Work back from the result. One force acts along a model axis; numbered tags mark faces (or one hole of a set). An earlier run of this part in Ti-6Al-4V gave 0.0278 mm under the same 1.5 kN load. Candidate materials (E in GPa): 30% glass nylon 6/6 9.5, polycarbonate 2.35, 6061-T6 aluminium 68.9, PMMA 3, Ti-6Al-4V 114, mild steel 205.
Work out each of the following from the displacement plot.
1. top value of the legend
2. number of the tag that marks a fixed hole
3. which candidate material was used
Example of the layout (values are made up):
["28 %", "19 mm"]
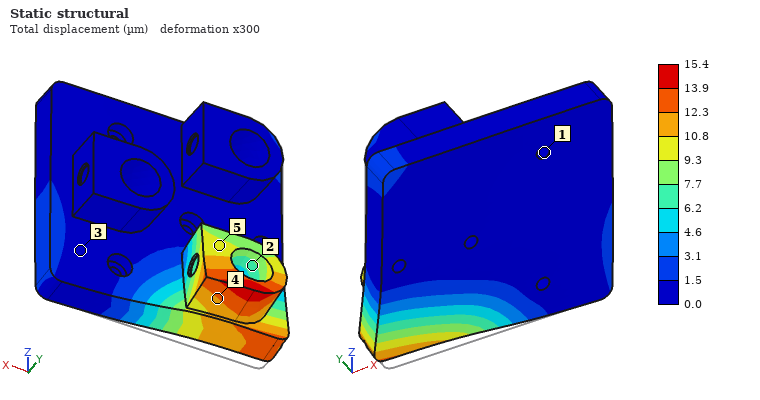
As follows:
["15.4 µm", "1", "mild steel"]
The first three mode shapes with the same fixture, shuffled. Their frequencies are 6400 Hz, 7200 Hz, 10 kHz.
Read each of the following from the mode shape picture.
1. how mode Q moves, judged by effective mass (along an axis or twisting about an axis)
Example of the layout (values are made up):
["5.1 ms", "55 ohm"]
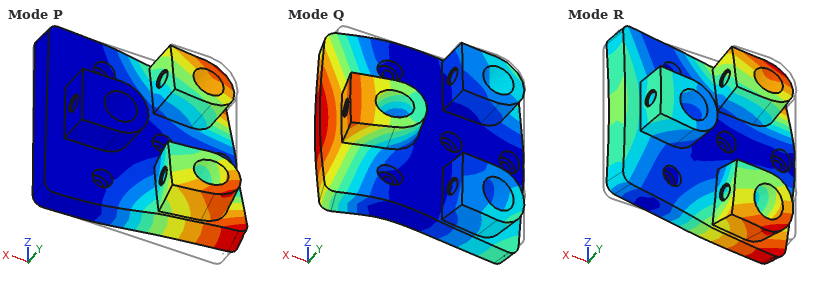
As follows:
["along Y"]
